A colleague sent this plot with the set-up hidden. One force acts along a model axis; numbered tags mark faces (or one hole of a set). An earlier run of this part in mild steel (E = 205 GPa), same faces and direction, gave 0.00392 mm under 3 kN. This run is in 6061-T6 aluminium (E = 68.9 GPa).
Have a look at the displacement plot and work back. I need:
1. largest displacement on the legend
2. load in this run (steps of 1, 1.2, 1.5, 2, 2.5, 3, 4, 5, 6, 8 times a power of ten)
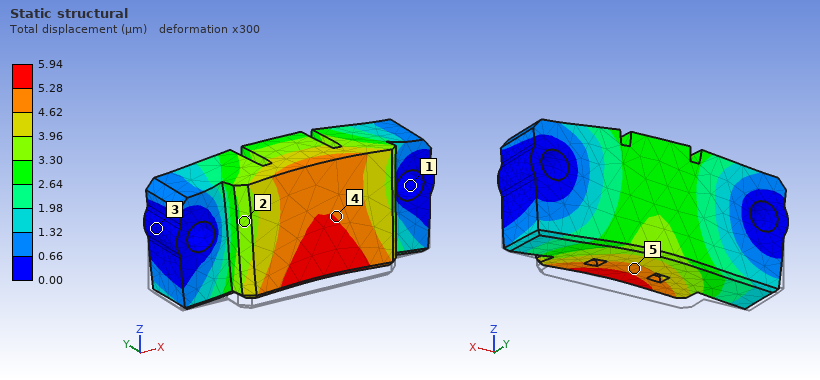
5.94 µm
1.5 kN
